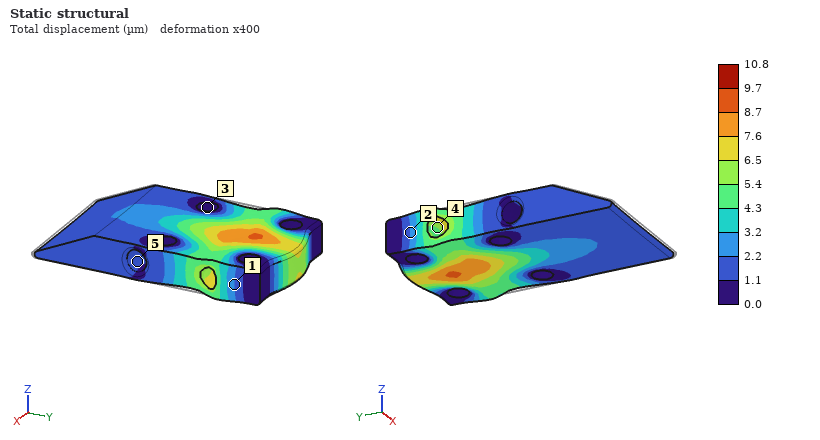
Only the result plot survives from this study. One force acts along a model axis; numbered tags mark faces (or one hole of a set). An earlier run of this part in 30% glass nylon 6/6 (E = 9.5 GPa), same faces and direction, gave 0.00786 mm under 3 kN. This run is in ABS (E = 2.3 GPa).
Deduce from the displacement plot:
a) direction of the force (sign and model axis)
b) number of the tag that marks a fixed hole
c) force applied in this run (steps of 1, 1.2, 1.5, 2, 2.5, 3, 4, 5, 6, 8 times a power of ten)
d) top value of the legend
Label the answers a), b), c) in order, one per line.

a) +Y
b) 3
c) 1 kN
d) 10.8 µm
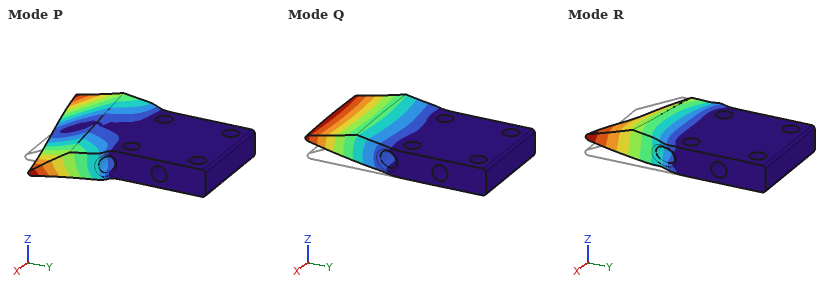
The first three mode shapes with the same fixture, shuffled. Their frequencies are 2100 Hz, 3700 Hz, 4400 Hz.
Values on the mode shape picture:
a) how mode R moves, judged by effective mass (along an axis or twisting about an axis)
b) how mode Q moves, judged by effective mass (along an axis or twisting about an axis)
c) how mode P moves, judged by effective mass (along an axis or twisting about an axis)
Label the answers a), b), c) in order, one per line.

a) along X
b) along Z
c) twisting about Y
